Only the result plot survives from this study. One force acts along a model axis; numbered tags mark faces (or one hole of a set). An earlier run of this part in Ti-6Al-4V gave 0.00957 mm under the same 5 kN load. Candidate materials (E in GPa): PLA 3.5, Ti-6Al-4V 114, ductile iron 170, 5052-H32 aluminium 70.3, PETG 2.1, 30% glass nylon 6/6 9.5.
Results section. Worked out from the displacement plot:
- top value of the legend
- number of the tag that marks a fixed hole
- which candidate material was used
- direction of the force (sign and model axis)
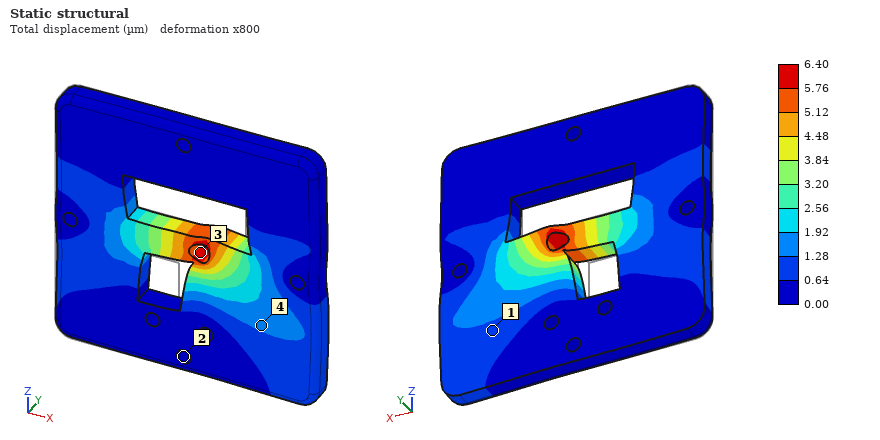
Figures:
6.40 µm
2
ductile iron
+X
